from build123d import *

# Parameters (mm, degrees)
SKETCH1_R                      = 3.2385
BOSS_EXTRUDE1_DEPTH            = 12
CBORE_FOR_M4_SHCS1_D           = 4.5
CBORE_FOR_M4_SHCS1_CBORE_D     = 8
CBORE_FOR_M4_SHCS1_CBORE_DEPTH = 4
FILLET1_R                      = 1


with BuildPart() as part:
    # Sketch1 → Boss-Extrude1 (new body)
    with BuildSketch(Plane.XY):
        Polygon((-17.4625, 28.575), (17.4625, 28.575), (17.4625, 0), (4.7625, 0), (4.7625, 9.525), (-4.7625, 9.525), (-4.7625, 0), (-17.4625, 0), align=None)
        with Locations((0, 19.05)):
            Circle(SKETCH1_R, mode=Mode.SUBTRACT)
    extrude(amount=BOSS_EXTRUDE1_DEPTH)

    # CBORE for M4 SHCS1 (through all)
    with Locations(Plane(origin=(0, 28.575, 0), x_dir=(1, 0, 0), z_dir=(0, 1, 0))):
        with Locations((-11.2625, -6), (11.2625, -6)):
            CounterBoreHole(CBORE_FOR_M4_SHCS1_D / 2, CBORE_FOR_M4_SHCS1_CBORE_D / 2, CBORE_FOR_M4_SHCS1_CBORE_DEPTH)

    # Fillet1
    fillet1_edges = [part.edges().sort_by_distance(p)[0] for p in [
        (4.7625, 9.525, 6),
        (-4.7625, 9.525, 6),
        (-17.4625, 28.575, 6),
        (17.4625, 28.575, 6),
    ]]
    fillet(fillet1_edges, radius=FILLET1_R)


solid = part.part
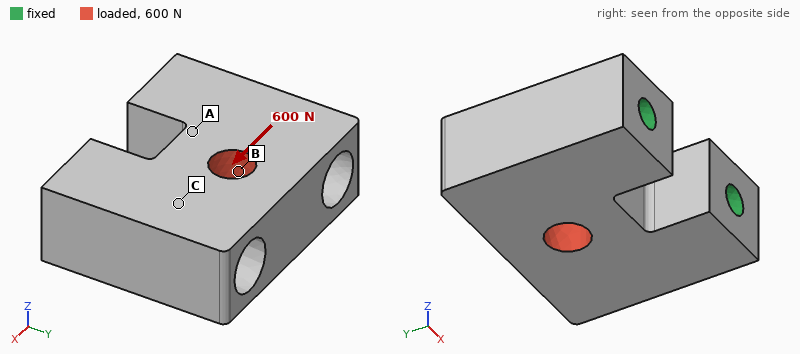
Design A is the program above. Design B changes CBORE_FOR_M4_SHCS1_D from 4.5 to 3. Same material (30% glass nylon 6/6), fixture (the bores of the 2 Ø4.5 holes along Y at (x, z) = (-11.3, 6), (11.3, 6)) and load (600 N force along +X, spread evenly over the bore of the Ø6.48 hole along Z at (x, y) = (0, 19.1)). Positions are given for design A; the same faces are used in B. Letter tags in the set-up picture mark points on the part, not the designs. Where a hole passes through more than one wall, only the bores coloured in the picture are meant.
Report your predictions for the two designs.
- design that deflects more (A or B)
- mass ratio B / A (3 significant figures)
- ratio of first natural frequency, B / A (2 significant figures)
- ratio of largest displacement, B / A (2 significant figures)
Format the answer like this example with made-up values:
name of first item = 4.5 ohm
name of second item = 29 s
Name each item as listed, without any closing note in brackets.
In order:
design that deflects more = B
mass ratio B / A = 1.05
ratio of first natural frequency, B / A = 0.86
ratio of largest displacement, B / A = 1.1
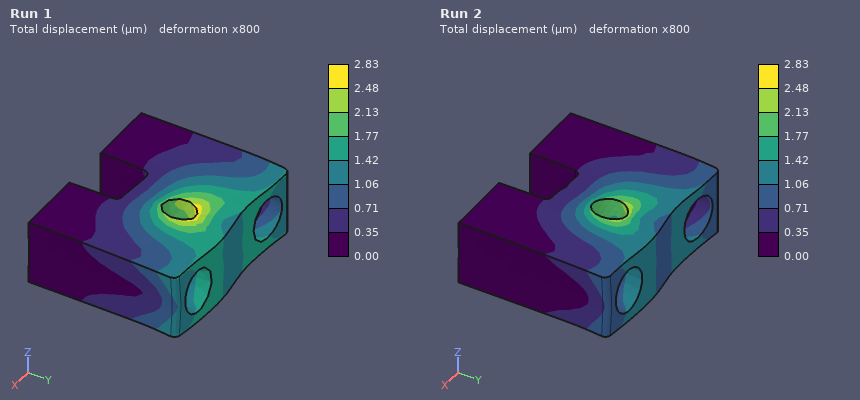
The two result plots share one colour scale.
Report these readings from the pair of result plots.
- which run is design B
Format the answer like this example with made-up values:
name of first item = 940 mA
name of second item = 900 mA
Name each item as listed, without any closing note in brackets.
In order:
which run is design B = Run 1
